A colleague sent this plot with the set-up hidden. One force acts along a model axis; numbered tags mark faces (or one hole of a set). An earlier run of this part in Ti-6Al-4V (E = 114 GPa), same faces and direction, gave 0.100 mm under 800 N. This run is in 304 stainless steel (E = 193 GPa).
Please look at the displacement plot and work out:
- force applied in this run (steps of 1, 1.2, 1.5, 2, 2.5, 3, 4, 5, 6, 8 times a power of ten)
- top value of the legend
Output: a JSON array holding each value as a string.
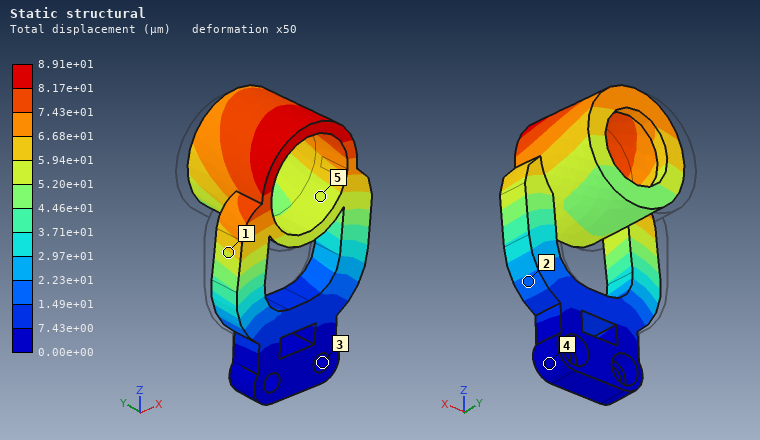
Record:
["1.2 kN", "8.91e+01 µm"]
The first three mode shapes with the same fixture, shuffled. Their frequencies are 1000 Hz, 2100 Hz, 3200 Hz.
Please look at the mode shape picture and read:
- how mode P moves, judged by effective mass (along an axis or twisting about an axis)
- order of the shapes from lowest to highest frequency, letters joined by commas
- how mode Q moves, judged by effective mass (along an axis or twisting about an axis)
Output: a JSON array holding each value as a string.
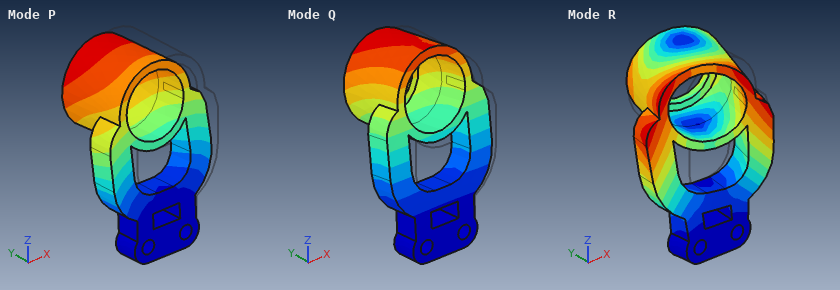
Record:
["along X", "Q, P, R", "along Y"]
